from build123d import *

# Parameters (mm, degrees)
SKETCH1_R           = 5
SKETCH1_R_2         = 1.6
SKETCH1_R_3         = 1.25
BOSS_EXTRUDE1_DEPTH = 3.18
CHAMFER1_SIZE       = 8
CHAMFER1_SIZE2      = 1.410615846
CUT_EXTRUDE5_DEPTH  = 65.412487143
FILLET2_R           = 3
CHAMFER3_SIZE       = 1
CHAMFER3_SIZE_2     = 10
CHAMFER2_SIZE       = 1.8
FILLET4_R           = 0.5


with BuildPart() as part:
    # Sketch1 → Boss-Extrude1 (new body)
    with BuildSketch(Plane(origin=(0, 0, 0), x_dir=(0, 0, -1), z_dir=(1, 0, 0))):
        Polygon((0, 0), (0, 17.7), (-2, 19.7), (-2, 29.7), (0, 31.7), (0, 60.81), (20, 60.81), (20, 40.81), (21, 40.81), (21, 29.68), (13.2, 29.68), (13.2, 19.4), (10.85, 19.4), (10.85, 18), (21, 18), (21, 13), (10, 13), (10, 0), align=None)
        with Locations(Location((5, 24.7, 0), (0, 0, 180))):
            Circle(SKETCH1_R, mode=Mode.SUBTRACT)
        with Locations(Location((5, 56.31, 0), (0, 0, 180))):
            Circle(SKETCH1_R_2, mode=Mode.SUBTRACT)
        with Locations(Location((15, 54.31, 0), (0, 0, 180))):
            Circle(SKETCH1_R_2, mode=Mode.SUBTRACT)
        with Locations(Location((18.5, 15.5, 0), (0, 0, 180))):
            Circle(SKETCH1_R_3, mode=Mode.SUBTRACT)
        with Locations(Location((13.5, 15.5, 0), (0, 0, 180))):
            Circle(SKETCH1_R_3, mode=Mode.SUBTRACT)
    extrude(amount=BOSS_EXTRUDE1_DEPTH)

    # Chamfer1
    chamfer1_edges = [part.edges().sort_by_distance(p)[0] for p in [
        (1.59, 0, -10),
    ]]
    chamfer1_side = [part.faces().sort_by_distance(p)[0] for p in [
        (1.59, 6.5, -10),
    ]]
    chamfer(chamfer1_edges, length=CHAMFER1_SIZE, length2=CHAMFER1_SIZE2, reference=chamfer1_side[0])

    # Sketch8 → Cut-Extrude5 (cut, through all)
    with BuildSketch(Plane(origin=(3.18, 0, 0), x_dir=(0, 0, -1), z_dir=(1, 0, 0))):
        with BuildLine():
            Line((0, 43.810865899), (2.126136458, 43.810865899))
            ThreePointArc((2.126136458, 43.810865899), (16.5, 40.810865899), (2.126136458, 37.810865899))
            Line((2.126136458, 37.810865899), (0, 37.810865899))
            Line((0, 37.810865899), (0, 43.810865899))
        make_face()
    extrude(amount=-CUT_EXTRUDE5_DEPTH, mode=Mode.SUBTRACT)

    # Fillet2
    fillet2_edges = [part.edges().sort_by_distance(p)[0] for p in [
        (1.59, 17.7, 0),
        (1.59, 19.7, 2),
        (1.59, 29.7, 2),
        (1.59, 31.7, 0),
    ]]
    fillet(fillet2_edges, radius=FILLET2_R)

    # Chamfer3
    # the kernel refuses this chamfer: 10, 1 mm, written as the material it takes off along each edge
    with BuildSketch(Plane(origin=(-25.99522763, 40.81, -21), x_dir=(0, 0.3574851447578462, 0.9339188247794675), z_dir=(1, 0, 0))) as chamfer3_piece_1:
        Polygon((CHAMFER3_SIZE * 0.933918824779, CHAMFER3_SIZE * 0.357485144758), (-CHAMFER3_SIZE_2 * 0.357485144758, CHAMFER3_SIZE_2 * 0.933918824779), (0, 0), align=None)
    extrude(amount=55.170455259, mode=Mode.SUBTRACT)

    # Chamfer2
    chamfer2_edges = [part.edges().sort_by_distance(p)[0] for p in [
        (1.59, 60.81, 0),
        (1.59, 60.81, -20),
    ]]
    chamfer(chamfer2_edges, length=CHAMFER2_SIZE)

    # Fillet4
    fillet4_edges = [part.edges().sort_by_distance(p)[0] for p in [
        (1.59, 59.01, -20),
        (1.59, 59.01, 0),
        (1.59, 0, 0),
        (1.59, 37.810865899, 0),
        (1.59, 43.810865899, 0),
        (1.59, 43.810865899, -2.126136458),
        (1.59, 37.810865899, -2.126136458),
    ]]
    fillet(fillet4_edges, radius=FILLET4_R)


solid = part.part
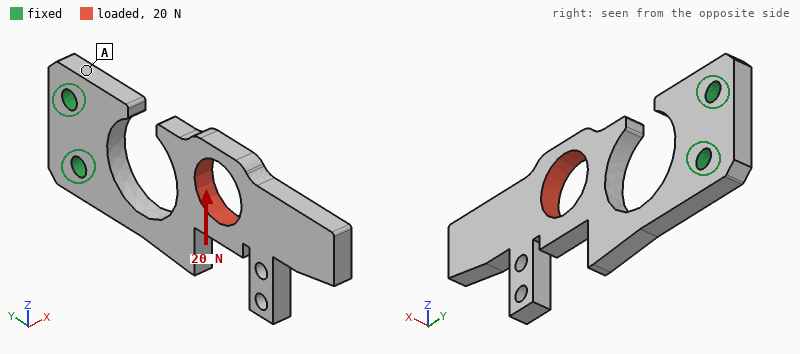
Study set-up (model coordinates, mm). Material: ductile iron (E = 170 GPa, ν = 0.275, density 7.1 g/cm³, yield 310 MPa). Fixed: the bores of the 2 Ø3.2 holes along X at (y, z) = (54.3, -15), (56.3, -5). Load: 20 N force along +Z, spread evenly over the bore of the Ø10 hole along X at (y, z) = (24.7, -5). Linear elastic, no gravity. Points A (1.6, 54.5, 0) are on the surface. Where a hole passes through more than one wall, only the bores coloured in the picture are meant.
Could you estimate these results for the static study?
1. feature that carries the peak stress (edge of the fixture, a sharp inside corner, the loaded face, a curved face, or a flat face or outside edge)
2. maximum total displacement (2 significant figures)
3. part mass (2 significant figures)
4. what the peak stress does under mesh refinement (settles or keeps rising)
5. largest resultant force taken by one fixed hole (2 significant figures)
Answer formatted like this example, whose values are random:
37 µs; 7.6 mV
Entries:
a sharp inside corner; 75 µm; 17 g; keeps rising; 49 N
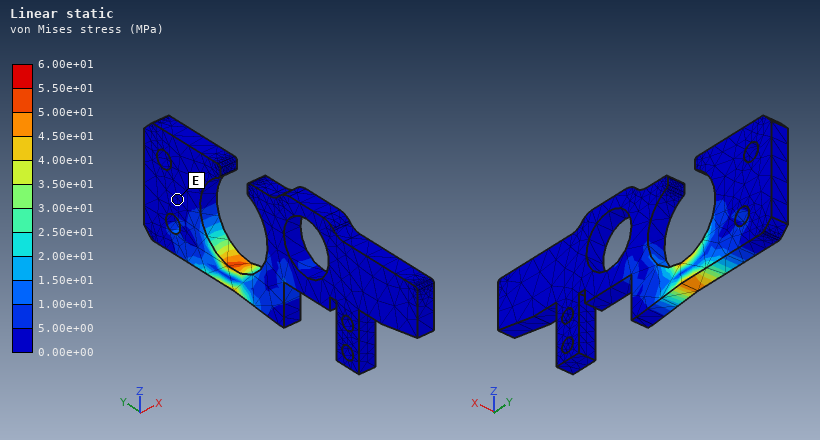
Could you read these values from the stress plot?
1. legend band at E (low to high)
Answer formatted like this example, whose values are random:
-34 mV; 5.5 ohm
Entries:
0.00e+00 to 5.00e+00 MPa
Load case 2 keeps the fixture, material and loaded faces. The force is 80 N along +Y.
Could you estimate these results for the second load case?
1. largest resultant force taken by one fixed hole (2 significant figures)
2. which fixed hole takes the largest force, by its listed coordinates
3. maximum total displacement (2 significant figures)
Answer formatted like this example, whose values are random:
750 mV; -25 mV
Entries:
74 N; (56.3, -5); 0.23 mm
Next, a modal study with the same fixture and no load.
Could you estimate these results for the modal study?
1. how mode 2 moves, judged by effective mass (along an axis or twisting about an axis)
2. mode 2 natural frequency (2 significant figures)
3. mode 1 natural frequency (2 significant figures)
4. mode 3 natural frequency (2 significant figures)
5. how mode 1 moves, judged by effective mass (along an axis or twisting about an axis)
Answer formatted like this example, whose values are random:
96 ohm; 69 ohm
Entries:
along Z; 830 Hz; 570 Hz; 2400 Hz; along X
